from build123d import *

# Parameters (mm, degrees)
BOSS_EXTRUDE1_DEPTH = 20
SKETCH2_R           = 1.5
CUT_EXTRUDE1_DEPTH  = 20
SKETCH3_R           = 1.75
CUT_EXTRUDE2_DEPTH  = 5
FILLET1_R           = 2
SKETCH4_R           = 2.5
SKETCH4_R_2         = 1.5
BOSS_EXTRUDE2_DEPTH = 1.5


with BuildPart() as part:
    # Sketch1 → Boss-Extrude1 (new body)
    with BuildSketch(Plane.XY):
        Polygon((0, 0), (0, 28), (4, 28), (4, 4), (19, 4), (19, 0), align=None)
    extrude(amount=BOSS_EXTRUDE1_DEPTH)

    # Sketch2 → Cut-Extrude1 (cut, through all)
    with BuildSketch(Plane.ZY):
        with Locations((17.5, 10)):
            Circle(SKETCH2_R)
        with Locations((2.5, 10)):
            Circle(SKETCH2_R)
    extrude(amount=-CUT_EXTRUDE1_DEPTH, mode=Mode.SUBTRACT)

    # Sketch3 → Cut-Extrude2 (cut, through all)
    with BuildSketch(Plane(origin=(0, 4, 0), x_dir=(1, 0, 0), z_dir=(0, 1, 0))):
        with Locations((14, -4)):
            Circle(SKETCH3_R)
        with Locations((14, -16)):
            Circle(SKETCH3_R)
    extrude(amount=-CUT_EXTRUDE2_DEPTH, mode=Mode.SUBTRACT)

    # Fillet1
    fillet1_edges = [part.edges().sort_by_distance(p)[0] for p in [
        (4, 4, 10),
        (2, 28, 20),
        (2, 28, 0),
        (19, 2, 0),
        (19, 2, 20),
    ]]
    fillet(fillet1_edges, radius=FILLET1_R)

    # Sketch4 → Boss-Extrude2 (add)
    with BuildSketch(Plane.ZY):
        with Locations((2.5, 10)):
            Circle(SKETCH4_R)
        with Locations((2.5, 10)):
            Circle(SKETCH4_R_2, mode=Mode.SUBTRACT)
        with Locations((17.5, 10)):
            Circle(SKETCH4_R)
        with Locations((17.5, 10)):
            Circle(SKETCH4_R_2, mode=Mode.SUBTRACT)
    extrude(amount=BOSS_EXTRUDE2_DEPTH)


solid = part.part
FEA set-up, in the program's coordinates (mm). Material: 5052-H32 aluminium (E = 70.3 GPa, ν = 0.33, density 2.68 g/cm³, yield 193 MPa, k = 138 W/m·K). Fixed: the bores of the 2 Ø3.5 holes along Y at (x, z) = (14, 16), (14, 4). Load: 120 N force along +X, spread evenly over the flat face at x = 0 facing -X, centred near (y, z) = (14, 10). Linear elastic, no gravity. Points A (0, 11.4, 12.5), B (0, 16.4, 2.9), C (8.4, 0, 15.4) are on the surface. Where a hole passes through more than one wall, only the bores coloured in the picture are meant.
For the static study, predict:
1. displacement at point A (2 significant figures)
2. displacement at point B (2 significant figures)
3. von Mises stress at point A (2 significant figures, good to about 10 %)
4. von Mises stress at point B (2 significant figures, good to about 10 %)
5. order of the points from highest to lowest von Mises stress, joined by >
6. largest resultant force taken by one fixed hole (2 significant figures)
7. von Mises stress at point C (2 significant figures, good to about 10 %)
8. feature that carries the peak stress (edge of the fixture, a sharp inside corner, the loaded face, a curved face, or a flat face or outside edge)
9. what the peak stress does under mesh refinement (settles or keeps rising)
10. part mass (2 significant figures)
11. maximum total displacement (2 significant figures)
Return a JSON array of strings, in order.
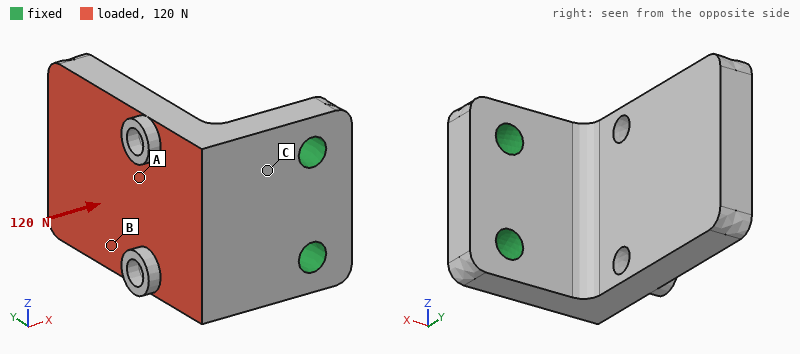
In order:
["29 µm", "42 µm", "12 MPa", "5.8 MPa", "C > A > B", "63 N", "24 MPa", "edge of the fixture", "keeps rising", "9.0 g", "78 µm"]
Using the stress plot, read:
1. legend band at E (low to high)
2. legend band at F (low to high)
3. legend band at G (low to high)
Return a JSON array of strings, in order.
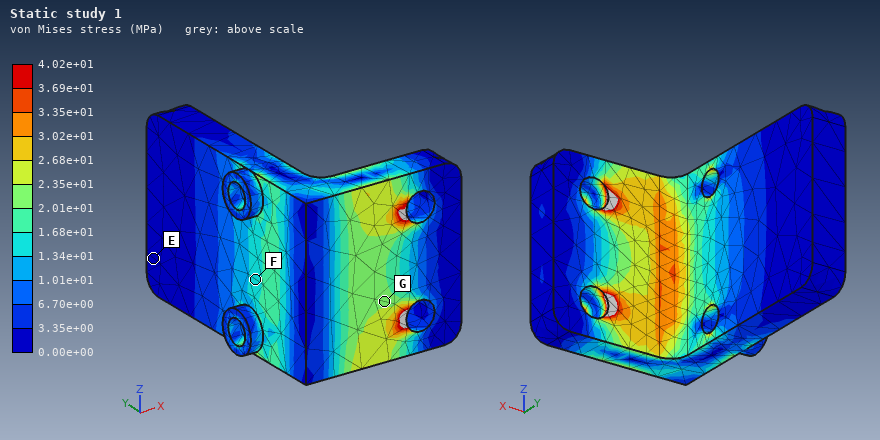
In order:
["0.00e+00 to 3.35e+00 MPa", "1.34e+01 to 1.68e+01 MPa", "2.01e+01 to 2.35e+01 MPa"]
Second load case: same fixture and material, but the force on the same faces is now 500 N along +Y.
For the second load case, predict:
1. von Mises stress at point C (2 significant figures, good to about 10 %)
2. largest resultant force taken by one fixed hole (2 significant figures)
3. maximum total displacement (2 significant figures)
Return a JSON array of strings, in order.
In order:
["75 MPa", "250 N", "0.17 mm"]
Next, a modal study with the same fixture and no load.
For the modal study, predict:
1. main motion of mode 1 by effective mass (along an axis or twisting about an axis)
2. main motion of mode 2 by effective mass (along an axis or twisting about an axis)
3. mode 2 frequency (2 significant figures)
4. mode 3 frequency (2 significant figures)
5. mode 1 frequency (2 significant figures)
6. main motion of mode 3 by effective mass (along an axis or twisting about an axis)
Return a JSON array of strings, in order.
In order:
["along X", "along Z", "5800 Hz", "11 kHz", "3100 Hz", "along Y"]
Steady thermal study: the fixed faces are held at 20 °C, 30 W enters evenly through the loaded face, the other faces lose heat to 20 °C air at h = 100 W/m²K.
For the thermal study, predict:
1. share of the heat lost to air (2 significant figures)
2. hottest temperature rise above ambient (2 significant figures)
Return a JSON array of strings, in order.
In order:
["15 %", "52 K"]
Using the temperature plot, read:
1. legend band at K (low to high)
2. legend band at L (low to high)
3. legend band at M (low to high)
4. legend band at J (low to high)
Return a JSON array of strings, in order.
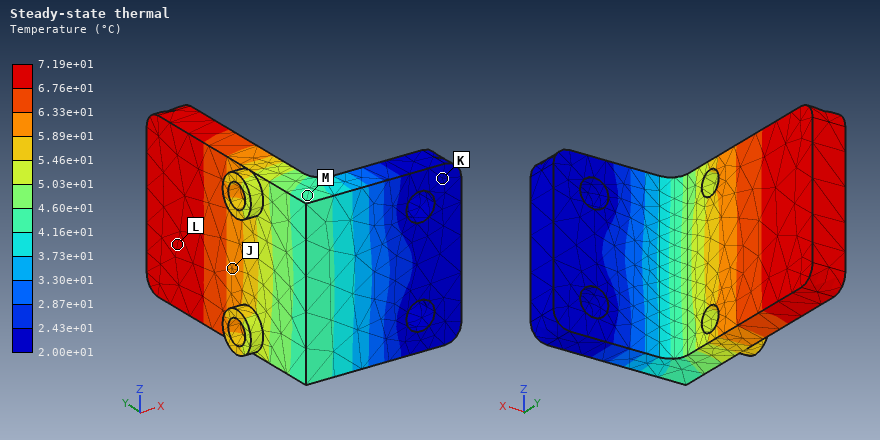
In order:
["2.00e+01 to 2.43e+01 °C", "6.76e+01 to 7.19e+01 °C", "4.16e+01 to 4.60e+01 °C", "5.89e+01 to 6.33e+01 °C"]
